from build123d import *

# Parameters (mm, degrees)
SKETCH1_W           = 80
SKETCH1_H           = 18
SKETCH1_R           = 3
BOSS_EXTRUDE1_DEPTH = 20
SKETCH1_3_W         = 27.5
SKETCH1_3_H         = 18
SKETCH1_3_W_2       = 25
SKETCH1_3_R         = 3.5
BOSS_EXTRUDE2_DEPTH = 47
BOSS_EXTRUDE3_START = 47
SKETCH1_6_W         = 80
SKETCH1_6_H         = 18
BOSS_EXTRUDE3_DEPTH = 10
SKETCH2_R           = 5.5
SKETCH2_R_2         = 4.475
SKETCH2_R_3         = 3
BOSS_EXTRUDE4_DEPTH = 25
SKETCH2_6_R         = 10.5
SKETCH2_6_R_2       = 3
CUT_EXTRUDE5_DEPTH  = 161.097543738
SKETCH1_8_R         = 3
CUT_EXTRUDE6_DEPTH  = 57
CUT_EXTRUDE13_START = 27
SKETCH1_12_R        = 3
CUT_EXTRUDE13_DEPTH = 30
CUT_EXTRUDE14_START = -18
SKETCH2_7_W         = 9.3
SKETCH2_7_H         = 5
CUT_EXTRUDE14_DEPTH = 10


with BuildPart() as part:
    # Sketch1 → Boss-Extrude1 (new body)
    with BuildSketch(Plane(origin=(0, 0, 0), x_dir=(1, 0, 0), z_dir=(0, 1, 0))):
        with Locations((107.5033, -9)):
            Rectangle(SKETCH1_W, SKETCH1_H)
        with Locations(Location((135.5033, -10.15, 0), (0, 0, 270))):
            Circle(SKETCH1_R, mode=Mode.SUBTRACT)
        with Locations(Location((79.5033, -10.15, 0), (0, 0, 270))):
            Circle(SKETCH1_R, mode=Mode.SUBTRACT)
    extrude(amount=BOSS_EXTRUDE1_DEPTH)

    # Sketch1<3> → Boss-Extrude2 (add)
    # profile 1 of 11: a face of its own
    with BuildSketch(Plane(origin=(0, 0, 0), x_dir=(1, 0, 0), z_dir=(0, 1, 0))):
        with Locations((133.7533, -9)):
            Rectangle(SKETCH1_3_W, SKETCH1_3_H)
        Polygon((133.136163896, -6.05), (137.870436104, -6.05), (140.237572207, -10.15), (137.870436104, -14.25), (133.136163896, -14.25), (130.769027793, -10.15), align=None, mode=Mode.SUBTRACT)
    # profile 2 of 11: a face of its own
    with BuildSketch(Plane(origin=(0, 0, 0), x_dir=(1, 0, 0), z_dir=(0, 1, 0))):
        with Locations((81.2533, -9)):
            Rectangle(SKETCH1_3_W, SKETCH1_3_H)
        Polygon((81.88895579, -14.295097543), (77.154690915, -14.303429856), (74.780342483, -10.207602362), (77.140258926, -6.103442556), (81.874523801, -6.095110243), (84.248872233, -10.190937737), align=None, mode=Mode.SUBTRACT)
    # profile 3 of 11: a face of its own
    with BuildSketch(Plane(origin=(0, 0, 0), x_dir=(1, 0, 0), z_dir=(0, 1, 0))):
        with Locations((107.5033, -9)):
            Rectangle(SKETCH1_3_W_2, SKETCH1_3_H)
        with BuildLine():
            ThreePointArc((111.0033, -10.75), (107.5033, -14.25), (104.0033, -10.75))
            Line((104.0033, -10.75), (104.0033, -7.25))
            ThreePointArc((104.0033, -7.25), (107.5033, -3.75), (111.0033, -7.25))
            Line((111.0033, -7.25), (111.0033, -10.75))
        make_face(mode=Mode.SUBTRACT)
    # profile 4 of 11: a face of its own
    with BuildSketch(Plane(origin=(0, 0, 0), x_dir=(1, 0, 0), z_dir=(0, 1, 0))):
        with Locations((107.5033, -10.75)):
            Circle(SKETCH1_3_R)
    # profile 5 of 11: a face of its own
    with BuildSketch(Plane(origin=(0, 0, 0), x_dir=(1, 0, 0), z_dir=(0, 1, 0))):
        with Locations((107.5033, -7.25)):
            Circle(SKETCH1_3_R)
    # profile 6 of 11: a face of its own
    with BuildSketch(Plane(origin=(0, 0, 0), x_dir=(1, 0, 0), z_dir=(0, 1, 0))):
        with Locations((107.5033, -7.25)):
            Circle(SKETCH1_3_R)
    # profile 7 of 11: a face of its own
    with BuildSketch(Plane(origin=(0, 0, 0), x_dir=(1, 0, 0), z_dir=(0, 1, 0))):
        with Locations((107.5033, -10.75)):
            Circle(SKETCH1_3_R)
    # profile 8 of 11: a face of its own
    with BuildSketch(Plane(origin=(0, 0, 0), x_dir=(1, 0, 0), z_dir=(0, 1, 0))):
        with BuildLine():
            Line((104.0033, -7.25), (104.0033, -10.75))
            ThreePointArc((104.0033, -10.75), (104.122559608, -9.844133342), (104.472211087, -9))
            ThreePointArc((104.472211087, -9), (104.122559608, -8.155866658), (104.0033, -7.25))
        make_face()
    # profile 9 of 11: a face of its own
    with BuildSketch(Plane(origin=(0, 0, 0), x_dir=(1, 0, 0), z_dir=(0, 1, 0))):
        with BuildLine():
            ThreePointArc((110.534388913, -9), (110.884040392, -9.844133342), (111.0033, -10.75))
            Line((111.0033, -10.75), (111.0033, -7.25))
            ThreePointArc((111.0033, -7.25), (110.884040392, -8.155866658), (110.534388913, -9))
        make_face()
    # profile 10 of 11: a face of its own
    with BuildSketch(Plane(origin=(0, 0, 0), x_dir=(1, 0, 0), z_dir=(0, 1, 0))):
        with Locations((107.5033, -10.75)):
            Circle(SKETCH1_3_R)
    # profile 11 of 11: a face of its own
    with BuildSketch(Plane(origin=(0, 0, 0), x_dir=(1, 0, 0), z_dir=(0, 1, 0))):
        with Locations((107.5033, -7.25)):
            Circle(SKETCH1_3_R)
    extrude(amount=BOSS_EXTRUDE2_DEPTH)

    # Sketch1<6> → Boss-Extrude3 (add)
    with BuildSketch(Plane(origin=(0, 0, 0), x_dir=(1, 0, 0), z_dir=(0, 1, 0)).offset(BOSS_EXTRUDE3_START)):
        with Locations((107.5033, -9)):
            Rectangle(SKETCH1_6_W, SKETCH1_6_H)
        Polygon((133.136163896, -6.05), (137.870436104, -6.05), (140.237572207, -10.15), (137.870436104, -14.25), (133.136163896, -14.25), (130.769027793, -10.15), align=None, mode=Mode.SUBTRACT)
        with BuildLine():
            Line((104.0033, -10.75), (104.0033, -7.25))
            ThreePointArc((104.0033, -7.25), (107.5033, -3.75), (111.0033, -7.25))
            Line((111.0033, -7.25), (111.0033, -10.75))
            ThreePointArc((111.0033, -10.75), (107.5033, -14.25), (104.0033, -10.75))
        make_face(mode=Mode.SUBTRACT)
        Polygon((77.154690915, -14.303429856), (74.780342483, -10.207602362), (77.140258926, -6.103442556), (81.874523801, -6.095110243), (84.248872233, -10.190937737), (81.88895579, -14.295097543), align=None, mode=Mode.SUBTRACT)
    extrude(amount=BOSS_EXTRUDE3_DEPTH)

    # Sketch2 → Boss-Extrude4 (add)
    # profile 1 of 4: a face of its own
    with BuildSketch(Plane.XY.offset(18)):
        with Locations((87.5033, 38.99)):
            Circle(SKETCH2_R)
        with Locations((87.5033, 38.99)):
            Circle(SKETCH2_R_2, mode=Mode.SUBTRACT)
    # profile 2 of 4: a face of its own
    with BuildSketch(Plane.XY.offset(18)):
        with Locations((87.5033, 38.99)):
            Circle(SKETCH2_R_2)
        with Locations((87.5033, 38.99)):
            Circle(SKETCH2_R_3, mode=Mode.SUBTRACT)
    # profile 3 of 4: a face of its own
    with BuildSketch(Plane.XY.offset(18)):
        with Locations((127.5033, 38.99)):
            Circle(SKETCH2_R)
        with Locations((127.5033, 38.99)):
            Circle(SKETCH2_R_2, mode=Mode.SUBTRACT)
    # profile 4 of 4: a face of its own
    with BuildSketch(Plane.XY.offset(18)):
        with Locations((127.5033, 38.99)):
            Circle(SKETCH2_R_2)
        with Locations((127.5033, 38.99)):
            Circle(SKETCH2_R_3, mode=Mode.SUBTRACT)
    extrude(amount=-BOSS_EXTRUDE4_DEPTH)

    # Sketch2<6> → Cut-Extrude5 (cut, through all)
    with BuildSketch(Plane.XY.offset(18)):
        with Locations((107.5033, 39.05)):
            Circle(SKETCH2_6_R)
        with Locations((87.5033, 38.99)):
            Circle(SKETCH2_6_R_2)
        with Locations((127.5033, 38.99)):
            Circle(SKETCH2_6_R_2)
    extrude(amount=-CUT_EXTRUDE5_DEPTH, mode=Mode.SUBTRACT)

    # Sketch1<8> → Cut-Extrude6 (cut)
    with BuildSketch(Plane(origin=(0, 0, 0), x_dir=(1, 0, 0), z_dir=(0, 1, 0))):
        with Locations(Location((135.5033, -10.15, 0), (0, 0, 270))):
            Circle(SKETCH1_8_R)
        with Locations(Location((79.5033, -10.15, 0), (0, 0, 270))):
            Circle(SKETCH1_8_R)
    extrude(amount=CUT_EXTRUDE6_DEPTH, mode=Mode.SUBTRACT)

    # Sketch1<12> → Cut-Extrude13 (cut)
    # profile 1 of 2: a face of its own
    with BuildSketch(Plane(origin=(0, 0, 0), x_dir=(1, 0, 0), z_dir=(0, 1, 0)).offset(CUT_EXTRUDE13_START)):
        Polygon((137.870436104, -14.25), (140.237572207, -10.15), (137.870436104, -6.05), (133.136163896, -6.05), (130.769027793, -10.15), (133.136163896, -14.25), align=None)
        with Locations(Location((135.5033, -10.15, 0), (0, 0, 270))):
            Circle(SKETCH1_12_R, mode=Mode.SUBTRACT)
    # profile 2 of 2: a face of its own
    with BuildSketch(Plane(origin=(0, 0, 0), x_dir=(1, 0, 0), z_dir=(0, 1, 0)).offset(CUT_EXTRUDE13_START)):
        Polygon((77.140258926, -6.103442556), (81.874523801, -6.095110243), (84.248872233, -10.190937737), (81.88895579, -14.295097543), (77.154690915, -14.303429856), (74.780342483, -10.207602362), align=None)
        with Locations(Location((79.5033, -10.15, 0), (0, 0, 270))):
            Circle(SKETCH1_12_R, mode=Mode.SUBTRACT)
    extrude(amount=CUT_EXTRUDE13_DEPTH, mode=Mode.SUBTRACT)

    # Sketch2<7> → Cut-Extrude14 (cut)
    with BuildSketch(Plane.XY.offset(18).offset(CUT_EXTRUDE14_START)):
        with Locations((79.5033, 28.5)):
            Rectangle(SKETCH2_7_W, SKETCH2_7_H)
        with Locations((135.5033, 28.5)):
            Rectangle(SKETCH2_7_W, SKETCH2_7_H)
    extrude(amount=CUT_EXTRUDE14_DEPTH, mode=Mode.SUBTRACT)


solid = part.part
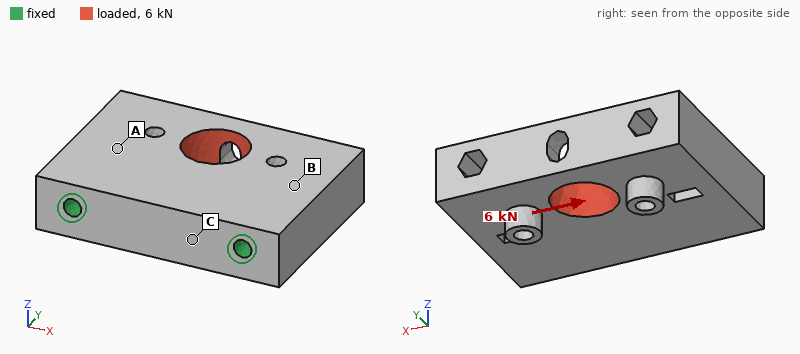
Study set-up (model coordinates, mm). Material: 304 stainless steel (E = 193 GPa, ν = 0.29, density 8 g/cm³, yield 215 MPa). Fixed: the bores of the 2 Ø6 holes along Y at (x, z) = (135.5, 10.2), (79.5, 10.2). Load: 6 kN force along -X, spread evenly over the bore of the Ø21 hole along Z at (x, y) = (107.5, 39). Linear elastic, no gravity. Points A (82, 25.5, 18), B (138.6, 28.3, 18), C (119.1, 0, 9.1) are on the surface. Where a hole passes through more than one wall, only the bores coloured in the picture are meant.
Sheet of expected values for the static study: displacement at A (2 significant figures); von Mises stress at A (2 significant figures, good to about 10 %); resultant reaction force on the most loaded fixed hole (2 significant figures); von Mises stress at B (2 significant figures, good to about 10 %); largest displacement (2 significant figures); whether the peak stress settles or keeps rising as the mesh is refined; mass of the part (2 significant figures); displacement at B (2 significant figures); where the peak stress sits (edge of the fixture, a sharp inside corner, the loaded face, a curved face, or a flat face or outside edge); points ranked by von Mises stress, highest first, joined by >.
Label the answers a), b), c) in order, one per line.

a) 1.2 µm
b) 11 MPa
c) 3.9 kN
d) 8.1 MPa
e) 5.1 µm
f) keeps rising
g) 550 g
h) 1.7 µm
i) edge of the fixture
j) A > B > C
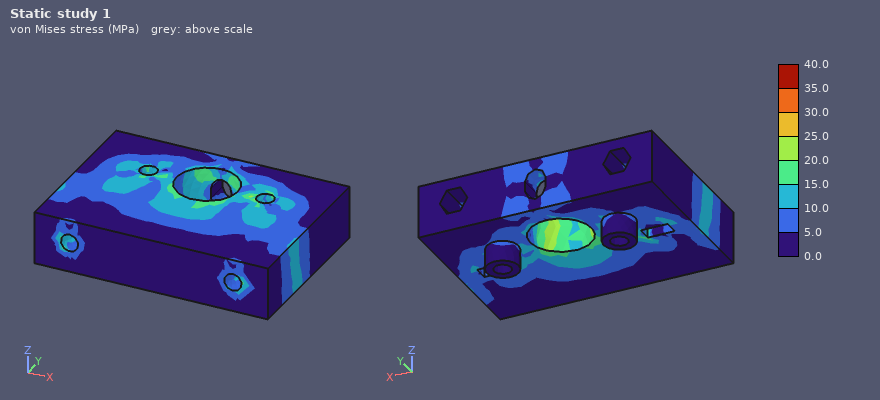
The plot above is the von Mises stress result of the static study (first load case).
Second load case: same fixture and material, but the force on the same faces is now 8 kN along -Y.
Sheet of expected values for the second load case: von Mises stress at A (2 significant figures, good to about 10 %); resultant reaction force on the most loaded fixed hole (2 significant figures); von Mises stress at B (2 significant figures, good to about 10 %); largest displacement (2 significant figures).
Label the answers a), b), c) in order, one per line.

a) 11 MPa
b) 4.2 kN
c) 6.2 MPa
d) 4.8 µm
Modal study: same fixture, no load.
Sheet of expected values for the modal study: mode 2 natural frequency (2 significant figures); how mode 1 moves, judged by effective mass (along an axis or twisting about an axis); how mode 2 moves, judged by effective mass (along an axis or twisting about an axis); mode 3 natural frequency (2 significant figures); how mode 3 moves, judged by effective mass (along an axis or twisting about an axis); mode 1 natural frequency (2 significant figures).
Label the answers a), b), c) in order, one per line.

a) 7900 Hz
b) along Z
c) twisting about Y
d) 11 kHz
e) along X
f) 4900 Hz
